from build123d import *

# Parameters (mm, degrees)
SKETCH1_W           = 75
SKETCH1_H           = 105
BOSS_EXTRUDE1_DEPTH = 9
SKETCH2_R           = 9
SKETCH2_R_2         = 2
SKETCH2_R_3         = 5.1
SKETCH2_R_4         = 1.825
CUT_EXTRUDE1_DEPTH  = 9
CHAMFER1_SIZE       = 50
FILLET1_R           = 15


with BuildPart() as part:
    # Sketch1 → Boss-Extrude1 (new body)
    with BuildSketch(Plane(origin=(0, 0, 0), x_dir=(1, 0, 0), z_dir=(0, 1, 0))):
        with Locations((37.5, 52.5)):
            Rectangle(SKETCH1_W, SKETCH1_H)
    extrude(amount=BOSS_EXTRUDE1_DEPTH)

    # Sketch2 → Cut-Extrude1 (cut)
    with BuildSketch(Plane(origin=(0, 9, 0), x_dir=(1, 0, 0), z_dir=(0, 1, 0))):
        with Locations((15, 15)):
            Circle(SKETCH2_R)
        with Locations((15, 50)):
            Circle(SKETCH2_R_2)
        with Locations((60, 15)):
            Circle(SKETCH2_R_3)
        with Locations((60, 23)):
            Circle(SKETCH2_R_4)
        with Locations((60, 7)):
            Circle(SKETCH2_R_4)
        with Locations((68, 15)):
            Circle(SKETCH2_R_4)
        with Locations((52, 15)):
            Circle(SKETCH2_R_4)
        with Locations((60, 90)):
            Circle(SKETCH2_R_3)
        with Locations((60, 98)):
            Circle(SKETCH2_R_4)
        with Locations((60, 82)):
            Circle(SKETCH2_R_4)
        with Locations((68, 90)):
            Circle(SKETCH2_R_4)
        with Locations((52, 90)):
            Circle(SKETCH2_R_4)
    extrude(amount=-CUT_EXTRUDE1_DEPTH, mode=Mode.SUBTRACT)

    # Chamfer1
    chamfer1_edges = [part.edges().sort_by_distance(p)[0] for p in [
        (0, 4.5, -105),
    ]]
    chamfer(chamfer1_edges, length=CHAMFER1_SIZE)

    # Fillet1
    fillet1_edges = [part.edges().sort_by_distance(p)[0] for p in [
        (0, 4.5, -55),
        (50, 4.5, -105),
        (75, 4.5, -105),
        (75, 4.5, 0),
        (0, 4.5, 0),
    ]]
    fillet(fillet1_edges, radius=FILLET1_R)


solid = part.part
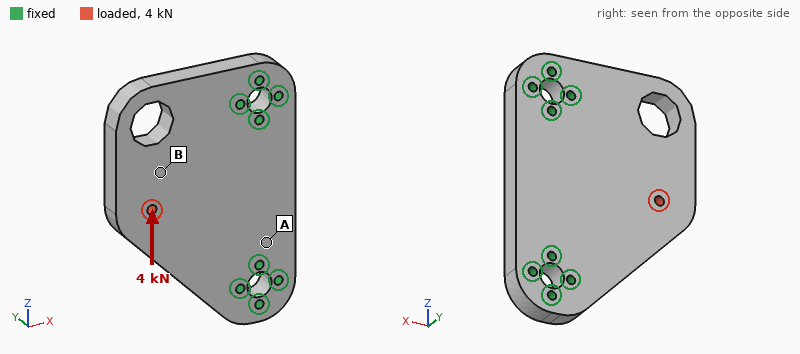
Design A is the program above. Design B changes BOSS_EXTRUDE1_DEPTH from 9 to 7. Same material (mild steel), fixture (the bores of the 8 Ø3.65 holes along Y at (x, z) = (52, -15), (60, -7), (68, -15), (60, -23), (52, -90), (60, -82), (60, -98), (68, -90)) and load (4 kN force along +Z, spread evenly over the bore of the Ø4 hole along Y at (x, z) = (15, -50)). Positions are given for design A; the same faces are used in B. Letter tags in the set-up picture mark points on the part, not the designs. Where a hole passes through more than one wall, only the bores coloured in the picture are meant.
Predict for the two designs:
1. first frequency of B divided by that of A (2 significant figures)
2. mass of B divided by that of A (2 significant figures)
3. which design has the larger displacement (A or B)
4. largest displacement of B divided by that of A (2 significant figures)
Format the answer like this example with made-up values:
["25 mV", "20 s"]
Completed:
["0.80", "0.78", "B", "1.3"]
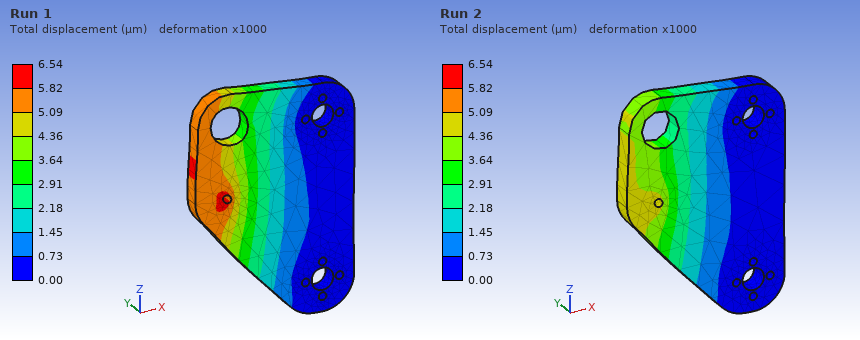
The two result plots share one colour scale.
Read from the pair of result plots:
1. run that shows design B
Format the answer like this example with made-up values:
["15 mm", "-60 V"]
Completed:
["Run 1"]
